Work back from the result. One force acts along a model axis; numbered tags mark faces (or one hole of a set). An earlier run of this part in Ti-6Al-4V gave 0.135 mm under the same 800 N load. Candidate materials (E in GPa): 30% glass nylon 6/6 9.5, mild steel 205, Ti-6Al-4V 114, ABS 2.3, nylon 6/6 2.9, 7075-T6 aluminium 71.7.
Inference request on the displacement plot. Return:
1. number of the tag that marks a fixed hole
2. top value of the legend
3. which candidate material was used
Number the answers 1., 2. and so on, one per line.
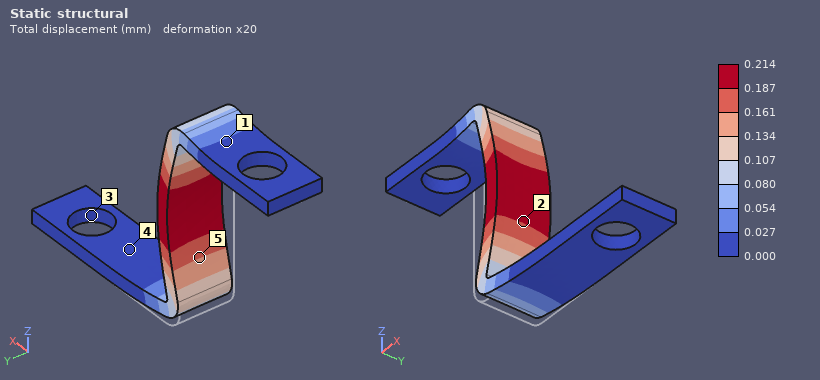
1. 3
2. 0.214 mm
3. 7075-T6 aluminium
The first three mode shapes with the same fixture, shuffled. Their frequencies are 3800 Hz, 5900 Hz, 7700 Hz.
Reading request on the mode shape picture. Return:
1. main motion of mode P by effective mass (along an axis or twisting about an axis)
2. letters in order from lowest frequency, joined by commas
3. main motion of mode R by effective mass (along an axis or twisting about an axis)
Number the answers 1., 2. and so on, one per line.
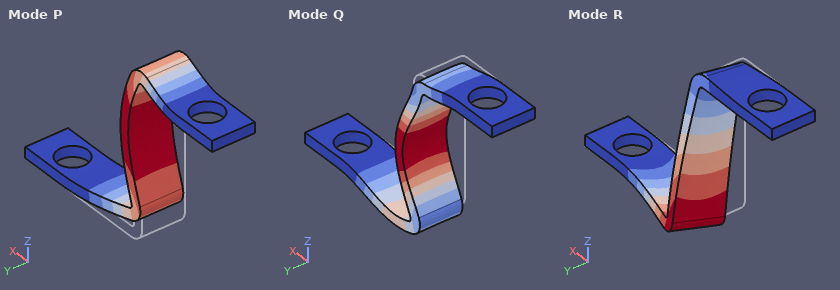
1. along Z
2. P, R, Q
3. along Y
